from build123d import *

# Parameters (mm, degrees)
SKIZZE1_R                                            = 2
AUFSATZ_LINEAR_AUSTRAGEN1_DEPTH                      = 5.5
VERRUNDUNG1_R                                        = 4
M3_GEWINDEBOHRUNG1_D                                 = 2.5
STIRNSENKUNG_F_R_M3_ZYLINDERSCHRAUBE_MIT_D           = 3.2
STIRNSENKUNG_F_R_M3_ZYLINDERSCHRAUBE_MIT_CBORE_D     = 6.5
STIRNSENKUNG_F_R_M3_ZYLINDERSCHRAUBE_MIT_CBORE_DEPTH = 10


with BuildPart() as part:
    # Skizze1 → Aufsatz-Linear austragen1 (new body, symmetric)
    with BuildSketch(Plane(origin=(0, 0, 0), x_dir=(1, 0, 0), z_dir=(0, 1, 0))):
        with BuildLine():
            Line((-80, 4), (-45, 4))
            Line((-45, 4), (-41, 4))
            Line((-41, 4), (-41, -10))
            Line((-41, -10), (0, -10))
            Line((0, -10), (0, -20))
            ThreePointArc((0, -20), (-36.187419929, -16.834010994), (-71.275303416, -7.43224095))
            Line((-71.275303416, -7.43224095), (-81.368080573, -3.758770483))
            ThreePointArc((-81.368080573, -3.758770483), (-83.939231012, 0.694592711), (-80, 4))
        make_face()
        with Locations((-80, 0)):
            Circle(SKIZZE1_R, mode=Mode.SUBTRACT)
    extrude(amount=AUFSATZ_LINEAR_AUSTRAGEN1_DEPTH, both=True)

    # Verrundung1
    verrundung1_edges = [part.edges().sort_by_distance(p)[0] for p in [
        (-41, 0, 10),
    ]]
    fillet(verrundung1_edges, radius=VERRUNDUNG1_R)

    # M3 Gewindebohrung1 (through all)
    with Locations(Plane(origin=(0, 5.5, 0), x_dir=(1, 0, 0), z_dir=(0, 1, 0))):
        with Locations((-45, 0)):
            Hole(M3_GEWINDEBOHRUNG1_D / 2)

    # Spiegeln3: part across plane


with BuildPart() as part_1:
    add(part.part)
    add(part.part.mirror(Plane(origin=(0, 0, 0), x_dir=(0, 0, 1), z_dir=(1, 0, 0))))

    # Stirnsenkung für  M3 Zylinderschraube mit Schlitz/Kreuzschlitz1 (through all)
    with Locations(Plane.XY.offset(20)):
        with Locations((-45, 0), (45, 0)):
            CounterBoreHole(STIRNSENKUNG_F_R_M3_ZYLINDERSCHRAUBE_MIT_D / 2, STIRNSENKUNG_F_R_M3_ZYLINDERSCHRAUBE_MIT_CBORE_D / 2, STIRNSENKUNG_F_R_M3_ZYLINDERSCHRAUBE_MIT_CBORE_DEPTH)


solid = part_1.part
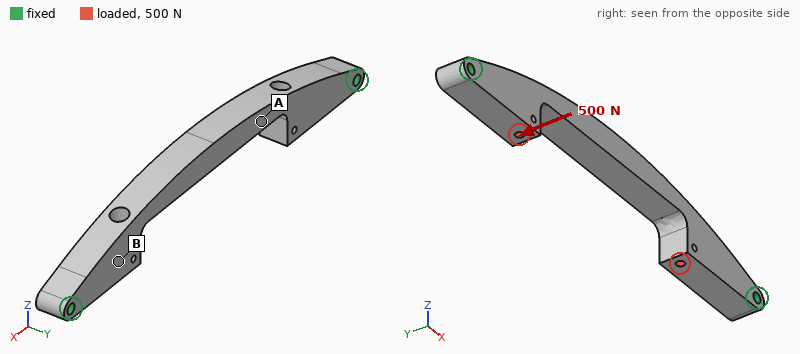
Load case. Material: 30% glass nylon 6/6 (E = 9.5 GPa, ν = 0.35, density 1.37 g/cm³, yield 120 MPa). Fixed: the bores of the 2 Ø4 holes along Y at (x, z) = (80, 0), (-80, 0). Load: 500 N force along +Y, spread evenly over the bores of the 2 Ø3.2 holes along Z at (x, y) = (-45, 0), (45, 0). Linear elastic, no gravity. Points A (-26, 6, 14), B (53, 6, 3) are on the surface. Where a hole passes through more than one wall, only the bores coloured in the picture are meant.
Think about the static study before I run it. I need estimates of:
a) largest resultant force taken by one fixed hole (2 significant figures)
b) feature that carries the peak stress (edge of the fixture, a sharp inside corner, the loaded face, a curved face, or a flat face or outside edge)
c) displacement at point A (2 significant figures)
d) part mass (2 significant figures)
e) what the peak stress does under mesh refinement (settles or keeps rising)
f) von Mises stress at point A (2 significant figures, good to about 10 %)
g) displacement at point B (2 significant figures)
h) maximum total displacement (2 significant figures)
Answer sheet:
250 N
edge of the fixture
0.36 mm
28 g
keeps rising
8.9 MPa
0.18 mm
0.42 mm
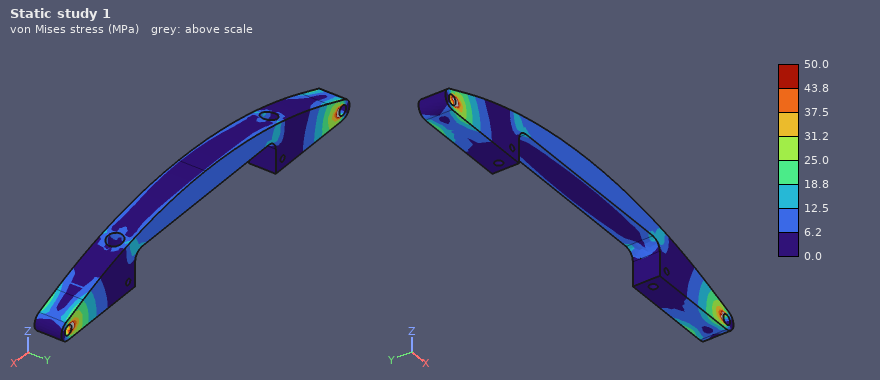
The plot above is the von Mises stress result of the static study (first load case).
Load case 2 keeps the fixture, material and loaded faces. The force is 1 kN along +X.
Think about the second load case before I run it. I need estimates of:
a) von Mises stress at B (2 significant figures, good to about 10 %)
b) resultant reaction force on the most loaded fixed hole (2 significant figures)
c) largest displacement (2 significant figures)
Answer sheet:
3.5 MPa
500 N
50 µm
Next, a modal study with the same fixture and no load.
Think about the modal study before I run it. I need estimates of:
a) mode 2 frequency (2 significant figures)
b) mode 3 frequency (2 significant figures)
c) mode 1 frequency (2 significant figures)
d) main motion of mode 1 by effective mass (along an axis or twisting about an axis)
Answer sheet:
1900 Hz
1900 Hz
1100 Hz
along Y
